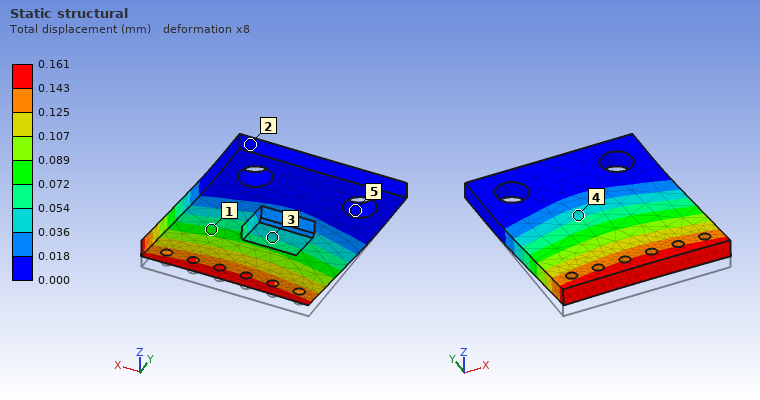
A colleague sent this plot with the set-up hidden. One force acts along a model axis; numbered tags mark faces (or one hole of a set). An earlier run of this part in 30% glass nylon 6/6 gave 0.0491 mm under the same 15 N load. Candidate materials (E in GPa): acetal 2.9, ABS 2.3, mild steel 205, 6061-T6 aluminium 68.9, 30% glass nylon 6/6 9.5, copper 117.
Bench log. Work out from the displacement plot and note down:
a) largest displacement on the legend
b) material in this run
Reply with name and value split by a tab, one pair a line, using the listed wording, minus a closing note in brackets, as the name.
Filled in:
largest displacement on the legend	0.161 mm
material in this run	acetal
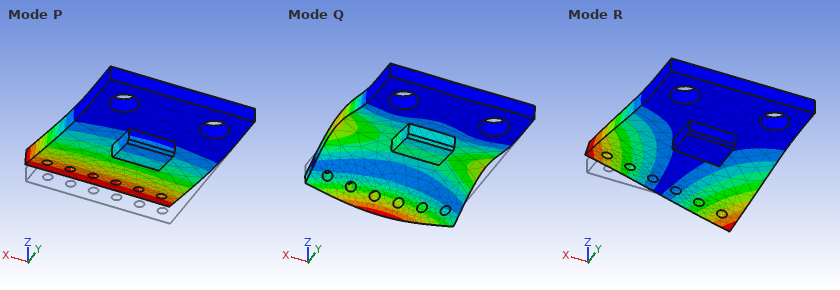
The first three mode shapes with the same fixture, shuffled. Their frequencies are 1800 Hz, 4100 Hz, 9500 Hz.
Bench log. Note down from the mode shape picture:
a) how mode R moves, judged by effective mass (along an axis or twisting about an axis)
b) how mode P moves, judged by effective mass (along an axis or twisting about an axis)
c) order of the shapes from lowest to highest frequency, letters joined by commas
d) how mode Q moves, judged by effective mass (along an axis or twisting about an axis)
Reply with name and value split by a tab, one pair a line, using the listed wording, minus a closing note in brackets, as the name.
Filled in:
how mode R moves, judged by effective mass	twisting about Y
how mode P moves, judged by effective mass	along Z
order of the shapes from lowest to highest frequency, letters joined by commas	P, R, Q
how mode Q moves, judged by effective mass	along Z
